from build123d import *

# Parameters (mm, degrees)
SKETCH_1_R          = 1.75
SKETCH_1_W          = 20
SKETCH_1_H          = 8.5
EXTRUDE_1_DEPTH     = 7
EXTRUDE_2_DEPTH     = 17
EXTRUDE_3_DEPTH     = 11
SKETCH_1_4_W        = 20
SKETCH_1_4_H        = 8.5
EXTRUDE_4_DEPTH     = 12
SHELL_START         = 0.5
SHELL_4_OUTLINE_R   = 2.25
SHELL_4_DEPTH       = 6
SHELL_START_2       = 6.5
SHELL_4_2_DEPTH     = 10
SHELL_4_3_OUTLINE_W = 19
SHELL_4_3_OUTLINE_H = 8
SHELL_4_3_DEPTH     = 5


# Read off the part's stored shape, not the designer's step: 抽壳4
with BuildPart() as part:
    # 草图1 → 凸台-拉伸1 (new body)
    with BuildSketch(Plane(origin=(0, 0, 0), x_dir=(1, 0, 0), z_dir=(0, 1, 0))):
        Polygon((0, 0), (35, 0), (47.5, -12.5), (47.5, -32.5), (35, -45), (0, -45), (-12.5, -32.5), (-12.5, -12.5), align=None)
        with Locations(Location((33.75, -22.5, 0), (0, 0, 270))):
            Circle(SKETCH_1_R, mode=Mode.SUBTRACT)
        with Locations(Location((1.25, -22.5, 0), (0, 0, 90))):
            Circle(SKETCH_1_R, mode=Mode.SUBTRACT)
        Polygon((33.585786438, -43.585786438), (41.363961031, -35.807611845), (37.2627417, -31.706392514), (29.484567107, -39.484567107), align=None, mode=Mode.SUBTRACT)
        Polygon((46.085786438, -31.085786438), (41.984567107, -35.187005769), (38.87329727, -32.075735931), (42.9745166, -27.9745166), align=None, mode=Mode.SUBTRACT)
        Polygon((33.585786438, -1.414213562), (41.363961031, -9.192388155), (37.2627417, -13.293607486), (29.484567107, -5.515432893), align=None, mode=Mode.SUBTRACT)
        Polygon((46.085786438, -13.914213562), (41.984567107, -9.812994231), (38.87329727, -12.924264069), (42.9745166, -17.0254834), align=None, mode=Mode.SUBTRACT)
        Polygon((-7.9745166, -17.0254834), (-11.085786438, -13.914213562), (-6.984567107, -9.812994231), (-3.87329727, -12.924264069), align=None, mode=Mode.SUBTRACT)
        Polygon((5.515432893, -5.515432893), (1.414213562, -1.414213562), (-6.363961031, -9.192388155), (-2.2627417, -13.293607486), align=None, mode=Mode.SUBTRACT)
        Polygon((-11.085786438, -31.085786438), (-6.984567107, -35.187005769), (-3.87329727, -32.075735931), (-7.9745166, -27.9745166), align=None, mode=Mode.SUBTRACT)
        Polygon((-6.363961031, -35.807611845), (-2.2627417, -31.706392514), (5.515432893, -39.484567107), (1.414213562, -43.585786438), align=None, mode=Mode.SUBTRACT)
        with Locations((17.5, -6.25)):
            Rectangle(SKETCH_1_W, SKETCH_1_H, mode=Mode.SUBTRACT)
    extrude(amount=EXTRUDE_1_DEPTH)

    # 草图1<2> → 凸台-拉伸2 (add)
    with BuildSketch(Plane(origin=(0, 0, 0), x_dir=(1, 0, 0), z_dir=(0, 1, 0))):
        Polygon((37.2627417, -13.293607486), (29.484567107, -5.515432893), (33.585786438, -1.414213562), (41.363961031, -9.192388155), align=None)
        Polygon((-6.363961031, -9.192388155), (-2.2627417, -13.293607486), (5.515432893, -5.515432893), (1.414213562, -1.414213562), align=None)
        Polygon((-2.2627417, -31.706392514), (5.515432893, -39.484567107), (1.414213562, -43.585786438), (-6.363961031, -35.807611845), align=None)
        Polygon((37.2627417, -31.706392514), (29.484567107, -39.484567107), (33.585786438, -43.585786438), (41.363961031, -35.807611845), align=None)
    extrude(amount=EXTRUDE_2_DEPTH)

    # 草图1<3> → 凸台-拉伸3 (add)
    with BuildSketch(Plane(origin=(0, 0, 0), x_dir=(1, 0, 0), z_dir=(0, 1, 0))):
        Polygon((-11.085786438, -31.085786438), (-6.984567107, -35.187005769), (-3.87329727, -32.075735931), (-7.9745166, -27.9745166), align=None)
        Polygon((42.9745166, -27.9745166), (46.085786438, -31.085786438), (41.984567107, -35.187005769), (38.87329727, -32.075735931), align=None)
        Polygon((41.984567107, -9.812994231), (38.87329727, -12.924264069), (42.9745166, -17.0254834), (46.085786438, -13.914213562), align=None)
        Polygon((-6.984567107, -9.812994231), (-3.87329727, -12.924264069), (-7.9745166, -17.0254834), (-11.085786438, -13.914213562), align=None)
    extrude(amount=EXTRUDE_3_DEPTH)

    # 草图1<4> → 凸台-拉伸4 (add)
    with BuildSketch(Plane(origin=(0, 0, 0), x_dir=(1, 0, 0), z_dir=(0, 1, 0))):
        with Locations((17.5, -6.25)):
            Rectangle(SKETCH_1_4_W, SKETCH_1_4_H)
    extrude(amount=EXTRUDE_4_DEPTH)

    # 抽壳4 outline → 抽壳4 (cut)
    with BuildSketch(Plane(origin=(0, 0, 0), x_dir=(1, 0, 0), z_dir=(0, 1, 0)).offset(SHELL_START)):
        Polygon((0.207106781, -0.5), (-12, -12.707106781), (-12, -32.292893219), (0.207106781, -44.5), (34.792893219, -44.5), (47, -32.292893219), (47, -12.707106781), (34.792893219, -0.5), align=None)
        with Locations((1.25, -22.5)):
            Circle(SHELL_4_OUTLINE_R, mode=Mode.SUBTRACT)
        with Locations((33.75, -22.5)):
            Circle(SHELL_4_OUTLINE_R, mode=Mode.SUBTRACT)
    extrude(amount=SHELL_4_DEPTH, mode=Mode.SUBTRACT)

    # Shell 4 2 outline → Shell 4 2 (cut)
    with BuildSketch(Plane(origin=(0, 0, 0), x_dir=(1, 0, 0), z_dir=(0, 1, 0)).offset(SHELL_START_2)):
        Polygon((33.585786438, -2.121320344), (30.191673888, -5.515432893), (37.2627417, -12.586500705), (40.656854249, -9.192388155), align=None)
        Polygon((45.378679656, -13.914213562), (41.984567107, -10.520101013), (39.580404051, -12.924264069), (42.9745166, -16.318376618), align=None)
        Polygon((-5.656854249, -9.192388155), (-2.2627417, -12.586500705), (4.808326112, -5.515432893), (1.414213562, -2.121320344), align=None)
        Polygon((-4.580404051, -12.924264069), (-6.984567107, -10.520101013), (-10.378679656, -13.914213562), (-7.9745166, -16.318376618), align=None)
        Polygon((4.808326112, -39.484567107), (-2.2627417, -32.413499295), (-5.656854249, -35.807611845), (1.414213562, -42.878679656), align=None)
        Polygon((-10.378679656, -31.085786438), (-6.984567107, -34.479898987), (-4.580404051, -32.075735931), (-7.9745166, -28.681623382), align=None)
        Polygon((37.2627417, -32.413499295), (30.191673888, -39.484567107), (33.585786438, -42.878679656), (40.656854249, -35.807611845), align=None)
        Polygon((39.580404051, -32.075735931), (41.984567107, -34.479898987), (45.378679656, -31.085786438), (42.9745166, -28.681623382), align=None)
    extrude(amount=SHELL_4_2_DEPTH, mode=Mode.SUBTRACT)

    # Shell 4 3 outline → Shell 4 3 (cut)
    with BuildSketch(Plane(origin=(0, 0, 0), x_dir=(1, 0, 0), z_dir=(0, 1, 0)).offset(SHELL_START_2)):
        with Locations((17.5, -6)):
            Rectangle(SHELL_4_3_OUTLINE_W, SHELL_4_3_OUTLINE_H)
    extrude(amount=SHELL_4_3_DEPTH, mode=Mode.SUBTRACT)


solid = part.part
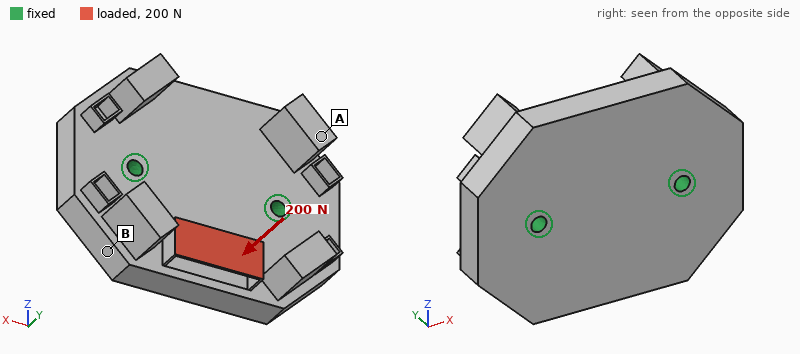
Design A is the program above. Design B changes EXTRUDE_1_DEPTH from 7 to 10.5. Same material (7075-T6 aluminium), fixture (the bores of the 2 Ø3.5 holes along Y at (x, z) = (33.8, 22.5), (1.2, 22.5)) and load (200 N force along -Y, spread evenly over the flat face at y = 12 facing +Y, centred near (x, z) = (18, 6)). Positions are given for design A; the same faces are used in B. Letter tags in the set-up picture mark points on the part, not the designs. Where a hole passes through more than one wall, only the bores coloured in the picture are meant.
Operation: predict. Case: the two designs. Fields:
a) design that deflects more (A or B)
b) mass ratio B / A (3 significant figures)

A
2.69
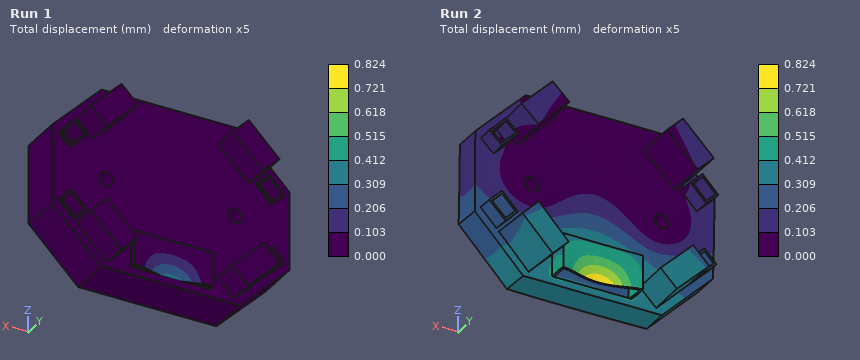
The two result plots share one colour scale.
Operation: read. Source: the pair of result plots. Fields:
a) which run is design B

Run 1
